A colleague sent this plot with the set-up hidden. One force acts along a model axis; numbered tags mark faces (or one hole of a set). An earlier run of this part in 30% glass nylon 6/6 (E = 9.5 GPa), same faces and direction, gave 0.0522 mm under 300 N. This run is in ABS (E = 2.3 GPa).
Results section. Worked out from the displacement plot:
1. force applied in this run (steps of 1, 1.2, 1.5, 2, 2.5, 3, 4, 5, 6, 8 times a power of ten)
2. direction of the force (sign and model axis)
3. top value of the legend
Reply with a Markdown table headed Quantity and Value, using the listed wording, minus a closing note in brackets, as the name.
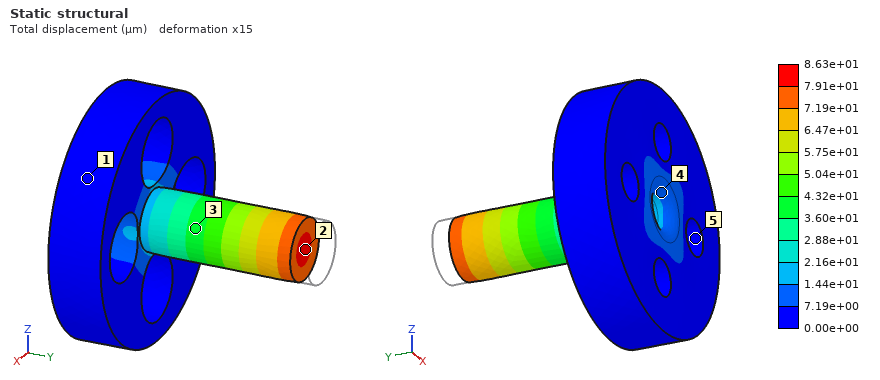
| Quantity | Value |
|---|---|
| force applied in this run | 120 N |
| direction of the force | -Y |
| top value of the legend | 8.63e+01 µm |
